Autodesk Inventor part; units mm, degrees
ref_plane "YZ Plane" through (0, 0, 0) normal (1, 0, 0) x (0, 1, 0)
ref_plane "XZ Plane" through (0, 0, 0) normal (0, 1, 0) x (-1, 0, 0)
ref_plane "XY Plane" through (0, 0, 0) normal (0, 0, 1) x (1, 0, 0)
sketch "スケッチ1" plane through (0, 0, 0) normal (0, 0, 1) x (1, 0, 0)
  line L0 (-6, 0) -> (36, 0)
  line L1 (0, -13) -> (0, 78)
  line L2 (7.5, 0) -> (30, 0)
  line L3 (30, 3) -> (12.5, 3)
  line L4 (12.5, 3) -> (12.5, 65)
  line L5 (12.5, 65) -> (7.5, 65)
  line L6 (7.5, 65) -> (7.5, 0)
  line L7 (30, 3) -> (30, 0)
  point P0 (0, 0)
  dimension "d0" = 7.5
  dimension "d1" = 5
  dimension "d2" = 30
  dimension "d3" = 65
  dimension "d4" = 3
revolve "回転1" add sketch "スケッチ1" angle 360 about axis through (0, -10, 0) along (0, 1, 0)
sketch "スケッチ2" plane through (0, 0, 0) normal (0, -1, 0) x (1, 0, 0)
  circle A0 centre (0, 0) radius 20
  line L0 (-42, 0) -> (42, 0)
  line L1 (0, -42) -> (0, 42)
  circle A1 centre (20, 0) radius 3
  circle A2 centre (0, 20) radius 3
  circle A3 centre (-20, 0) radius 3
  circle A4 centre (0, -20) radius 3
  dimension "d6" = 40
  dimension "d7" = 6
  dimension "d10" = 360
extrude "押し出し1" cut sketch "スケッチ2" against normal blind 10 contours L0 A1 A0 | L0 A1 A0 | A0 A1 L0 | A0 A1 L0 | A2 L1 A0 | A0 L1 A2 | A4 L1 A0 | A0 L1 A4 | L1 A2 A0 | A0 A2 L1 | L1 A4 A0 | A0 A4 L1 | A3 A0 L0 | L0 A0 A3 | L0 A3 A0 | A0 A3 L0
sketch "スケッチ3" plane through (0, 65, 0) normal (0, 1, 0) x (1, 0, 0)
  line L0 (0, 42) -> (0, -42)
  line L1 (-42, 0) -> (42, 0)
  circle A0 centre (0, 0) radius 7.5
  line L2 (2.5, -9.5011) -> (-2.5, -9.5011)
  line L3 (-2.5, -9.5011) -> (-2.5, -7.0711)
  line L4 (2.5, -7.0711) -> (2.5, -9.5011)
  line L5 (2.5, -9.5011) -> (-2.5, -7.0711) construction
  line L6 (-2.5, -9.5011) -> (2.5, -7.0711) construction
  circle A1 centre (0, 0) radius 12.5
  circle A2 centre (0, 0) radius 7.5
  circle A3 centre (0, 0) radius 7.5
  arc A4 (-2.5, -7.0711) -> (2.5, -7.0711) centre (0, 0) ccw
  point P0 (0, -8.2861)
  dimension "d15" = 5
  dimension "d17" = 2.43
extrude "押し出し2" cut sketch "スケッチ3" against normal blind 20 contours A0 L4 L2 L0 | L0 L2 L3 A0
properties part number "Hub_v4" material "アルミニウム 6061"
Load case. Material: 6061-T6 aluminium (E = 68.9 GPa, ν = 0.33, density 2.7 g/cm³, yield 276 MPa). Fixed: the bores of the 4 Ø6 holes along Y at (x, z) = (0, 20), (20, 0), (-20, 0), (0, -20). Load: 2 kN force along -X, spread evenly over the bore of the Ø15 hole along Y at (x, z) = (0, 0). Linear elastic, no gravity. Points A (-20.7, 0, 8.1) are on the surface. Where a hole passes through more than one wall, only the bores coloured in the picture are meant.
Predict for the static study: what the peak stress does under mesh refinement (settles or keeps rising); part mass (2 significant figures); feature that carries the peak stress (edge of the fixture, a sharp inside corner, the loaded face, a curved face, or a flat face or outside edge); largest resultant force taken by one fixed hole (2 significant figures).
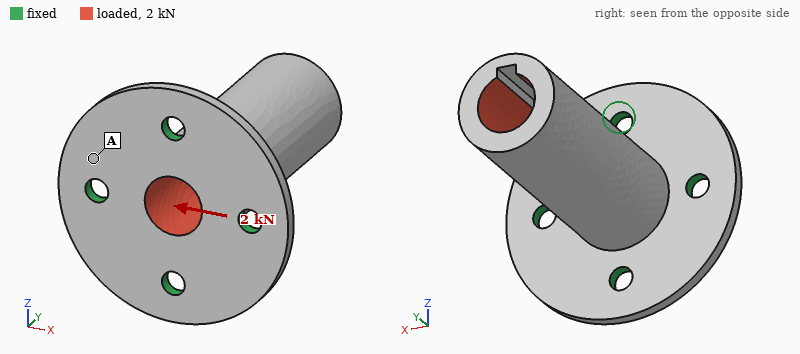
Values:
keeps rising
73 g
edge of the fixture
2.0 kN
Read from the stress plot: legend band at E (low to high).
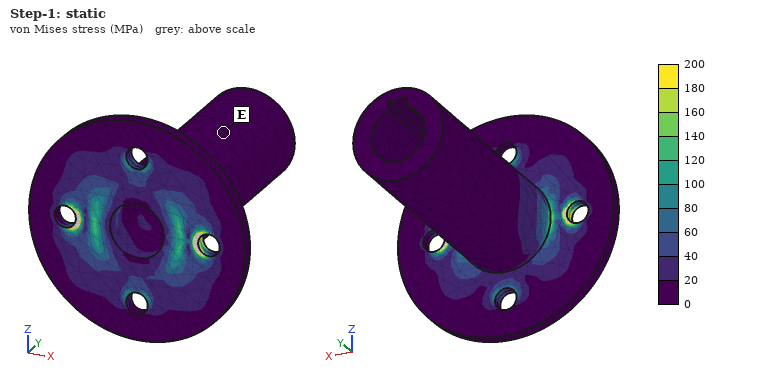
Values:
0 to 20 MPa
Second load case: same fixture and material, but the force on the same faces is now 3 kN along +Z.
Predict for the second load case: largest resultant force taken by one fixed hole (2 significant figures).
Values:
3.0 kN
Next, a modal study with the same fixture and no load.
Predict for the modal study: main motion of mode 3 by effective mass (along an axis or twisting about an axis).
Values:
along Y
